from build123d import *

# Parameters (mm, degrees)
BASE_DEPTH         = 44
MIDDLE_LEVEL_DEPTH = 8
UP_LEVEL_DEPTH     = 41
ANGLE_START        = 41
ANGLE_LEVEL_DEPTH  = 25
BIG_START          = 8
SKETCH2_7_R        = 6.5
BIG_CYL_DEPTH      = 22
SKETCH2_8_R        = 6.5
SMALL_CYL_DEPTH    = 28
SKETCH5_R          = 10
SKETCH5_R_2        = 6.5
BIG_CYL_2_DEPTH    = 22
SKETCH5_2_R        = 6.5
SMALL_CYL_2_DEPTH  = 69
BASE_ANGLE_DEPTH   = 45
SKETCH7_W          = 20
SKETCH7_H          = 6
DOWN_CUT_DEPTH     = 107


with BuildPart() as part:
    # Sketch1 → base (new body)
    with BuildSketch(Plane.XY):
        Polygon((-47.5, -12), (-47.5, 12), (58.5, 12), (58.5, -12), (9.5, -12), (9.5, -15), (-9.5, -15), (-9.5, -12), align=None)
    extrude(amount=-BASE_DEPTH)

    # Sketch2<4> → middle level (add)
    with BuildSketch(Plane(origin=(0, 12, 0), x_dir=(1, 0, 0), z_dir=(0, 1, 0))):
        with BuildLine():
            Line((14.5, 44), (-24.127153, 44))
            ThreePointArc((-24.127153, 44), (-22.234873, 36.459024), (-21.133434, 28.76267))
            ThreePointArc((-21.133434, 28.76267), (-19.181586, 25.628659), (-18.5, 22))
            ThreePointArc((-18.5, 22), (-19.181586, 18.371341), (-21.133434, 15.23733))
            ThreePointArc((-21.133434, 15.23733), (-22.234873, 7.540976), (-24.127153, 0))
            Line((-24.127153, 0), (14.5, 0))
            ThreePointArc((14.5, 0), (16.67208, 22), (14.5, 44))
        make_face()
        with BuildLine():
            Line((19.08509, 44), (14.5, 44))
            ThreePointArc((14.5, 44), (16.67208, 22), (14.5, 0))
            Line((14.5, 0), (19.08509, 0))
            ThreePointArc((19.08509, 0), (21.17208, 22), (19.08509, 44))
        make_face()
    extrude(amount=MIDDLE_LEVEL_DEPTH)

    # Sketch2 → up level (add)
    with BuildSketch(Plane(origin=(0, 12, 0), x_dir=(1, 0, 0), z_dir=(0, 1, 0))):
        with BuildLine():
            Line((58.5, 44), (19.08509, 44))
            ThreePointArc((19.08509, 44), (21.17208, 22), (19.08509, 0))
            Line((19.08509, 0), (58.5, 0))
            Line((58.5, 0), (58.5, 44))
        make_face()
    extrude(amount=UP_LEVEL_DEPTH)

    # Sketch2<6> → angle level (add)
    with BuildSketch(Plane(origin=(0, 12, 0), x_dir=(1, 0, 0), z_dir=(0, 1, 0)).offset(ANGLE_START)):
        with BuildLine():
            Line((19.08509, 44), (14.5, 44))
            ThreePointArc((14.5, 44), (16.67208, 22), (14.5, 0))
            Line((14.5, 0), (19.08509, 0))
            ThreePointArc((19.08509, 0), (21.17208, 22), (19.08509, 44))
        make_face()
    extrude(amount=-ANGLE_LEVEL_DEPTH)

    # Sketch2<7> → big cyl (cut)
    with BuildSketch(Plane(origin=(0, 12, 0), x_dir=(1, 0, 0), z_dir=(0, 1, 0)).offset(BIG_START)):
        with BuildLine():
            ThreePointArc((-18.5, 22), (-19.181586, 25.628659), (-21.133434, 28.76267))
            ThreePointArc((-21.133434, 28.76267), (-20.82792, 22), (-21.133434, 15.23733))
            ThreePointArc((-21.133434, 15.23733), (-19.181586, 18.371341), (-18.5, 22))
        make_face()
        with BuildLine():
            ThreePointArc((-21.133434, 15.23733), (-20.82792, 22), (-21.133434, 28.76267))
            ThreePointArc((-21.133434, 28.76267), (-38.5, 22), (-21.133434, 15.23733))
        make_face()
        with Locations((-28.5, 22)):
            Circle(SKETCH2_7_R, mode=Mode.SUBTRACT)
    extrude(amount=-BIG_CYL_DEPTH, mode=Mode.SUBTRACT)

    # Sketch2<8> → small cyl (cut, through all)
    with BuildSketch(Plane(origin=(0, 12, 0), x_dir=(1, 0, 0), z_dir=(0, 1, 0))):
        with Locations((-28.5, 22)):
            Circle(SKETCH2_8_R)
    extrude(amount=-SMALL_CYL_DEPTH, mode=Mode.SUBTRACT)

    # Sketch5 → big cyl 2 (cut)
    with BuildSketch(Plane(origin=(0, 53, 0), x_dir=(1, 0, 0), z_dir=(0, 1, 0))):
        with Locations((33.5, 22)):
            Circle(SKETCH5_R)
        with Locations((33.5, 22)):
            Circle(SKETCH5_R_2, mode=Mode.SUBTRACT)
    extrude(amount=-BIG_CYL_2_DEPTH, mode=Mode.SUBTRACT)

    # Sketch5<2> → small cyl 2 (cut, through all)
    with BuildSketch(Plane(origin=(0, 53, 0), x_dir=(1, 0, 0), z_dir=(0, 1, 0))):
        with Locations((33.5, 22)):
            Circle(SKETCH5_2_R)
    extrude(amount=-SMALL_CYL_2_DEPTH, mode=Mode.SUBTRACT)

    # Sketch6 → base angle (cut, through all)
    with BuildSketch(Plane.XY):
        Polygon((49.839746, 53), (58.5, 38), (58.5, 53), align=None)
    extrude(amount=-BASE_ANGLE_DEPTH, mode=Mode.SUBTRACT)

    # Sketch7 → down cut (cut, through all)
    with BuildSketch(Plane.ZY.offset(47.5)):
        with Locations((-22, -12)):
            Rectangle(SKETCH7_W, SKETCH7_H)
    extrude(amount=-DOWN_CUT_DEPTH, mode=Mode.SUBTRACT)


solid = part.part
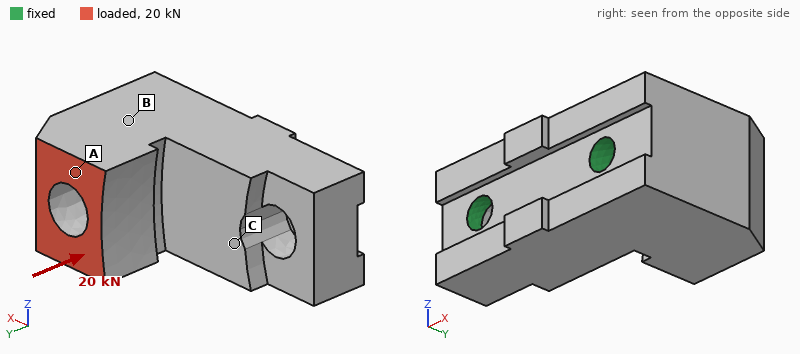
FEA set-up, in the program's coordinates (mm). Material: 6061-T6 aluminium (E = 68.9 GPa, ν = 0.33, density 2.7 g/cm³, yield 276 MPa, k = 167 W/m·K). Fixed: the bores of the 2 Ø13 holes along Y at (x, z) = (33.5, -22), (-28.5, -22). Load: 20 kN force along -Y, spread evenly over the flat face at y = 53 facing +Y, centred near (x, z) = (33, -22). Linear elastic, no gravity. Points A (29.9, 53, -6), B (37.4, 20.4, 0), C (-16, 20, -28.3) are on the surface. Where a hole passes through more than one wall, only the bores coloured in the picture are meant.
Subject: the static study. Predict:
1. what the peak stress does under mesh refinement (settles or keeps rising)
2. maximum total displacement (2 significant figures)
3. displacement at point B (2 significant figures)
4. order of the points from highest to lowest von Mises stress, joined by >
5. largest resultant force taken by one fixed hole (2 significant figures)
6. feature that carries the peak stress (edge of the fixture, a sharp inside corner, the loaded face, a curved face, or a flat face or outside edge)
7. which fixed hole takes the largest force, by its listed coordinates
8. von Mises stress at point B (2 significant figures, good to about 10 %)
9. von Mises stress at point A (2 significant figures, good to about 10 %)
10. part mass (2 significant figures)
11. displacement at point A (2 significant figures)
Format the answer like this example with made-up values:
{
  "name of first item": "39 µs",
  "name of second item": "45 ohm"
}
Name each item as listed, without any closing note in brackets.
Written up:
{
  "what the peak stress does under mesh refinement": "keeps rising",
  "maximum total displacement": "17 µm",
  "displacement at point B": "4.2 µm",
  "order of the points from highest to lowest von Mises stress, joined by >": "A > B > C",
  "largest resultant force taken by one fixed hole": "20 kN",
  "feature that carries the peak stress": "edge of the fixture",
  "which fixed hole takes the largest force, by its listed coordinates": "(33.5, -22)",
  "von Mises stress at point B": "9.2 MPa",
  "von Mises stress at point A": "18 MPa",
  "part mass": "470 g",
  "displacement at point A": "13 µm"
}
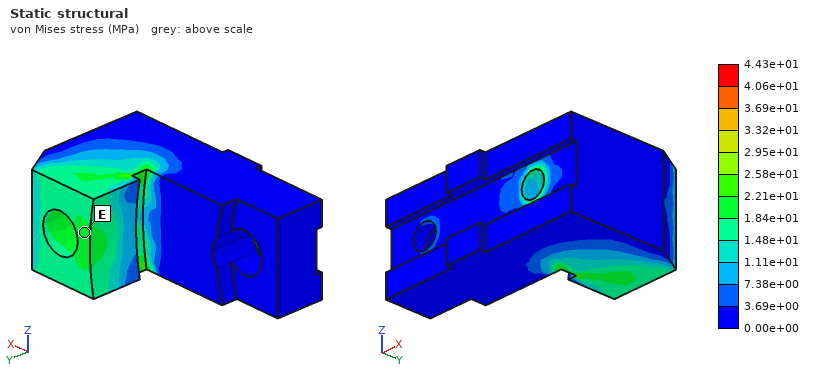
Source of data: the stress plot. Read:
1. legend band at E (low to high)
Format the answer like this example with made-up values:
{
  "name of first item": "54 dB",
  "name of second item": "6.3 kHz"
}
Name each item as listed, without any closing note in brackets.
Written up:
{
  "legend band at E": "1.84e+01 to 2.21e+01 MPa"
}
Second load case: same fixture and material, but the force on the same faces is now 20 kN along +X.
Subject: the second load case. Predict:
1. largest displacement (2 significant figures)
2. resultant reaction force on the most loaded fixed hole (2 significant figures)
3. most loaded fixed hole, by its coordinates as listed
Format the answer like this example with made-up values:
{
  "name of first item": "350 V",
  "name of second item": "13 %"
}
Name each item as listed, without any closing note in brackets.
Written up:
{
  "largest displacement": "86 µm",
  "resultant reaction force on the most loaded fixed hole": "19 kN",
  "most loaded fixed hole, by its coordinates as listed": "(33.5, -22)"
}
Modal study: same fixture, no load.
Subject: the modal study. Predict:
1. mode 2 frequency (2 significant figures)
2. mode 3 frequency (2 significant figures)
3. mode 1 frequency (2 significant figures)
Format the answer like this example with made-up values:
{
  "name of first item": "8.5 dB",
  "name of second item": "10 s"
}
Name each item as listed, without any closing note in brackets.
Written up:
{
  "mode 2 frequency": "13 kHz",
  "mode 3 frequency": "13 kHz",
  "mode 1 frequency": "10 kHz"
}
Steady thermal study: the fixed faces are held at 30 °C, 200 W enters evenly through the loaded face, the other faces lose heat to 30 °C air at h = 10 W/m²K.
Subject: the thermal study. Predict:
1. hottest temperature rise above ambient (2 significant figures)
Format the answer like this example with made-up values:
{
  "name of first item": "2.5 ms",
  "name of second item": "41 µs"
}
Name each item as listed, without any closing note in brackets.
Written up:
{
  "hottest temperature rise above ambient": "33 K"
}
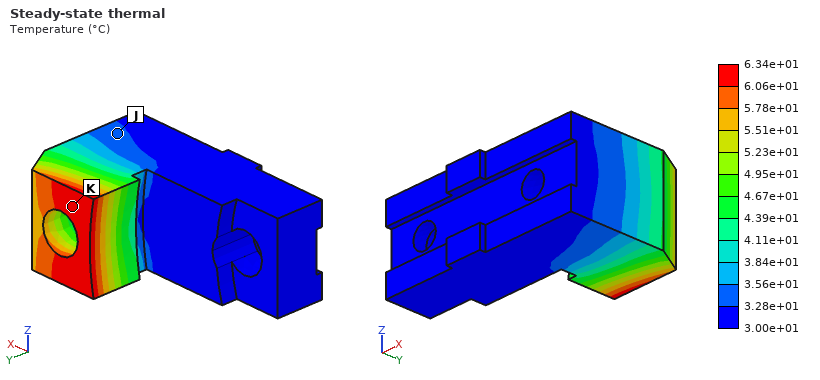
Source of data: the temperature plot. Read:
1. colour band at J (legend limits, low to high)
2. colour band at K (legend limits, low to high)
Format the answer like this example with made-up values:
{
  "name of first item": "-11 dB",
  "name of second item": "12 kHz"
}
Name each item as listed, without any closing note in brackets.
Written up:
{
  "colour band at J": "3.28e+01 to 3.56e+01 °C",
  "colour band at K": "6.06e+01 to 6.34e+01 °C"
}
